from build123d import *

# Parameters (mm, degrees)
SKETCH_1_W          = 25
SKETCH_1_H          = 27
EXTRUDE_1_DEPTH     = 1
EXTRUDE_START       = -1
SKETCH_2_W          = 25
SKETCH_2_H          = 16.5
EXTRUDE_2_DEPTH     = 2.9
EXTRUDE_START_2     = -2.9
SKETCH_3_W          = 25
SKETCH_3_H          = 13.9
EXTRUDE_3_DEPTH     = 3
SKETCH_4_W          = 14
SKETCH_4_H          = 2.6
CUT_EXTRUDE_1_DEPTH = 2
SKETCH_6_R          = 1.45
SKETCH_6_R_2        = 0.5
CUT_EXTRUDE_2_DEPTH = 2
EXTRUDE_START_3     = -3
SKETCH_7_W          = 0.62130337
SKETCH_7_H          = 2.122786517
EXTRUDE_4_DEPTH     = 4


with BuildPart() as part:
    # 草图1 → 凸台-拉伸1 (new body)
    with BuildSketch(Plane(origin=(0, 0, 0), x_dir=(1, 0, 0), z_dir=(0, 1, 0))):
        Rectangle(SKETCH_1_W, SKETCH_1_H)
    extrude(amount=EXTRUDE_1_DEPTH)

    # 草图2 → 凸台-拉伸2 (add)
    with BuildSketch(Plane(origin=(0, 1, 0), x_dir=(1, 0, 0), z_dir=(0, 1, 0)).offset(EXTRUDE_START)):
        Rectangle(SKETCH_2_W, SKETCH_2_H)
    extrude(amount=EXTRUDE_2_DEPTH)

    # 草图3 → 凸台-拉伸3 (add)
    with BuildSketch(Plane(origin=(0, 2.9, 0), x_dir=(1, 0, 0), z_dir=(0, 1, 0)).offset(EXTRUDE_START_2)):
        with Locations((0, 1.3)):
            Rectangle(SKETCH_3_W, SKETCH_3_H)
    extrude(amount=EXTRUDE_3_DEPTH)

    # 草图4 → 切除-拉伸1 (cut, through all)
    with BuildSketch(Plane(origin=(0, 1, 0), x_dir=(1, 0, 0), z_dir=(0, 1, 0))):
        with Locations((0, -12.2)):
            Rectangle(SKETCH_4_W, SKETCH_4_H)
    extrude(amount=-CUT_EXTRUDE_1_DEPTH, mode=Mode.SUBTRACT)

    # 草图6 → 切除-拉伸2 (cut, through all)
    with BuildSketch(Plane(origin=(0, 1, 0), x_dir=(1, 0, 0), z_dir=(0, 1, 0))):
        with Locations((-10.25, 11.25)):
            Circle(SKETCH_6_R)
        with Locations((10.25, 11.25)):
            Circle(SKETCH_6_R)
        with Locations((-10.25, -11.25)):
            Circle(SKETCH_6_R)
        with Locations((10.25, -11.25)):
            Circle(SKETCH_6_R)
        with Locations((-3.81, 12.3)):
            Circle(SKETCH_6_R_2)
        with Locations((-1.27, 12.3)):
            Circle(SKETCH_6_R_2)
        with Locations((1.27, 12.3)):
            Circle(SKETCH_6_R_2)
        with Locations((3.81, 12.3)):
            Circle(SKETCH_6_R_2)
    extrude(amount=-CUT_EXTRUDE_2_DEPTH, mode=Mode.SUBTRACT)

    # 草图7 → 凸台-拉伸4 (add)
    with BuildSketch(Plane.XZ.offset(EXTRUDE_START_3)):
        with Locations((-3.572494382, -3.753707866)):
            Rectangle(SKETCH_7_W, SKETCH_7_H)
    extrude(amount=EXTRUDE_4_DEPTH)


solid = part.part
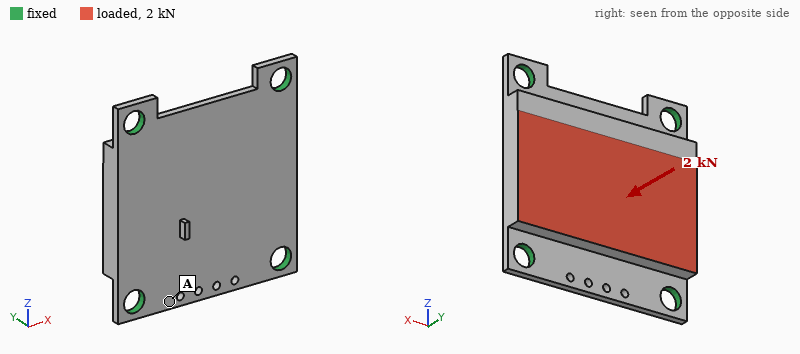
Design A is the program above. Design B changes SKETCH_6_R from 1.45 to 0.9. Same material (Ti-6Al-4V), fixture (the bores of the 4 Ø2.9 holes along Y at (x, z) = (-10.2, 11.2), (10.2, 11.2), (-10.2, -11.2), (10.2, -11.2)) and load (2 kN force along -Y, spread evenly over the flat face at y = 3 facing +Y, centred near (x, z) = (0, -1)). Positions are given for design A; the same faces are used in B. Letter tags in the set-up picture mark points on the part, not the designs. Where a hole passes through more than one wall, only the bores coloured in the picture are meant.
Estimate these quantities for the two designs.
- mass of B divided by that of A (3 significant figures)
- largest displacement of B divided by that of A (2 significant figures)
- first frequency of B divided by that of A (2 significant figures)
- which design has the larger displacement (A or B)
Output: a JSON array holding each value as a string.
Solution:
["1.01", "1.3", "0.85", "B"]
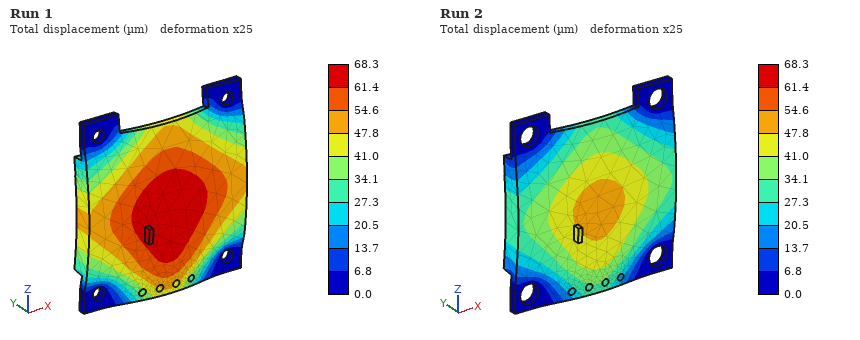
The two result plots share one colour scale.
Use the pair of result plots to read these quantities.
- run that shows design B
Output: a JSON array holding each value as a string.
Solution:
["Run 1"]
